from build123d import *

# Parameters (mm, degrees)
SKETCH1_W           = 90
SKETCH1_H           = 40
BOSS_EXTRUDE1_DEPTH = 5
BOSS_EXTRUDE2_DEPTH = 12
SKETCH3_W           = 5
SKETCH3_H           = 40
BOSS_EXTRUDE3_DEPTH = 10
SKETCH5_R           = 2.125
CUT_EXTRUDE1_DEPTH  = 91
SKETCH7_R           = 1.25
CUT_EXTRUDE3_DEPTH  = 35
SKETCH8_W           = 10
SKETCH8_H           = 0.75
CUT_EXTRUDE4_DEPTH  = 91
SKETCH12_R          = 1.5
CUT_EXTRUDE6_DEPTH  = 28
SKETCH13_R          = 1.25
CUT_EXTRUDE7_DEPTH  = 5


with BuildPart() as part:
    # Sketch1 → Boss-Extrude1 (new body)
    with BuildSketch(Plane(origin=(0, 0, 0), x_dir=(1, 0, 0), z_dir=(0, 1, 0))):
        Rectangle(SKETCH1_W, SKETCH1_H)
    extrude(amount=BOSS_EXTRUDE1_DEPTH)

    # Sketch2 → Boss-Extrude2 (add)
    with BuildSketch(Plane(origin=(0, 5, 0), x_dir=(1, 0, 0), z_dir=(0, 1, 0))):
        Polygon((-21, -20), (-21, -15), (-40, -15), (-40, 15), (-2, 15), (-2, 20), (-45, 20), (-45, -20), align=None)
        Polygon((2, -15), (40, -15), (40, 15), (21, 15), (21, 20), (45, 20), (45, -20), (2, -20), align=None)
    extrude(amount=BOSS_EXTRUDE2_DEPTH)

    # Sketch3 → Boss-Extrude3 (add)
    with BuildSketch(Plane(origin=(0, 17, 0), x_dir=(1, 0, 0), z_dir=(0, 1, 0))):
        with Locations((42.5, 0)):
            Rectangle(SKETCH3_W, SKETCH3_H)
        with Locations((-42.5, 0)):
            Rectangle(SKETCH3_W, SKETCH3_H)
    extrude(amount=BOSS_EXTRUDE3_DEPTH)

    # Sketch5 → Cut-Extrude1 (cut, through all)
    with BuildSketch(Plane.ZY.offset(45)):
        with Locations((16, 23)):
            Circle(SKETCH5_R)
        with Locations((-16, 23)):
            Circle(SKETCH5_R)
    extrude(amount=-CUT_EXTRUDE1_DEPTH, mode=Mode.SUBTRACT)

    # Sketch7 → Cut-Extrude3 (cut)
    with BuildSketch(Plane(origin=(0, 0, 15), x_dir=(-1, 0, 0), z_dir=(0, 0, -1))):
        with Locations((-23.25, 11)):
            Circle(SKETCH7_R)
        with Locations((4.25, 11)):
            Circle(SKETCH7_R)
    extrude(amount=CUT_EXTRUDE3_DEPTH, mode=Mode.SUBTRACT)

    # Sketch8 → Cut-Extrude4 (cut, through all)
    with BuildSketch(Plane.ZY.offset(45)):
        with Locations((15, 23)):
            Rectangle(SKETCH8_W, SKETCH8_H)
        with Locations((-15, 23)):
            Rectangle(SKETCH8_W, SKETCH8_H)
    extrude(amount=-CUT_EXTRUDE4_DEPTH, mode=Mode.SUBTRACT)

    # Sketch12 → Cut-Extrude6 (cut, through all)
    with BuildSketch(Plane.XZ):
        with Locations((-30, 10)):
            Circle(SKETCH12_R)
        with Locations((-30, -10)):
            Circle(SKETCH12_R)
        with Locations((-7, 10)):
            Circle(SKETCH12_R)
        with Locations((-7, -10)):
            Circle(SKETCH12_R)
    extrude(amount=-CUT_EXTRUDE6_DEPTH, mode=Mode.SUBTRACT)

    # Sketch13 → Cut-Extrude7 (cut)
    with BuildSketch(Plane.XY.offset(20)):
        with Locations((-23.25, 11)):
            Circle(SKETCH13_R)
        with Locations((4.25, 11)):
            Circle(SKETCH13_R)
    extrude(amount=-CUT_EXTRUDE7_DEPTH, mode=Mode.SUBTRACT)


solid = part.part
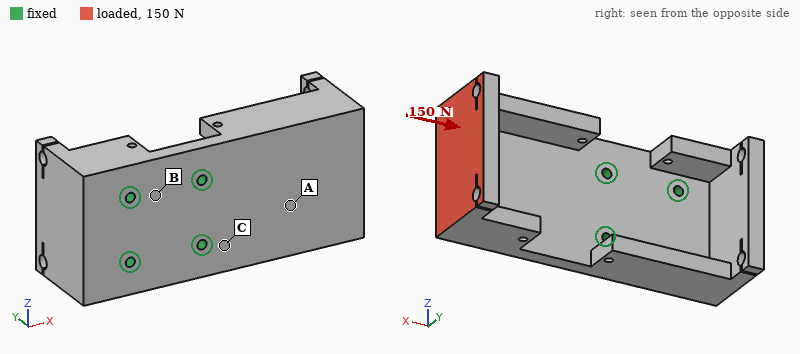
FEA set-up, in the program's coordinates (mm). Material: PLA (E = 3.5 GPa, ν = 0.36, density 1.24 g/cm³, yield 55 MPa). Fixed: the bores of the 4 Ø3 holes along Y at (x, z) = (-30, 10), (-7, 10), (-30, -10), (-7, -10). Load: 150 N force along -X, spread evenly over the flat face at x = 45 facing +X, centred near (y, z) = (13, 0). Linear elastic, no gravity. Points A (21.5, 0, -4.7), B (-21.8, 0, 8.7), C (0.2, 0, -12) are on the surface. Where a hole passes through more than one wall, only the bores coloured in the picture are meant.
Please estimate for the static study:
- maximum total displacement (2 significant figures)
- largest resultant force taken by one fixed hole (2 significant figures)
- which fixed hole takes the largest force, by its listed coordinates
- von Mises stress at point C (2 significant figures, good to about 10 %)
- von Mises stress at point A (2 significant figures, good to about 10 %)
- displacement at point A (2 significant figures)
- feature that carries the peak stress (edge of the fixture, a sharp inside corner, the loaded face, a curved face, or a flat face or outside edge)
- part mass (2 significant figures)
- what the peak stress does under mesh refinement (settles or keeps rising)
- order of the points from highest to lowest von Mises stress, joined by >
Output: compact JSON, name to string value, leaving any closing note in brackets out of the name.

{"maximum total displacement": "1.2 mm", "largest resultant force taken by one fixed hole": "65 N", "which fixed hole takes the largest force, by its listed coordinates": "(-7, 10)", "von Mises stress at point C": "6.8 MPa", "von Mises stress at point A": "3.0 MPa", "displacement at point A": "0.36 mm", "feature that carries the peak stress": "edge of the fixture", "part mass": "41 g", "what the peak stress does under mesh refinement": "keeps rising", "order of the points from highest to lowest von Mises stress, joined by >": "C > A > B"}
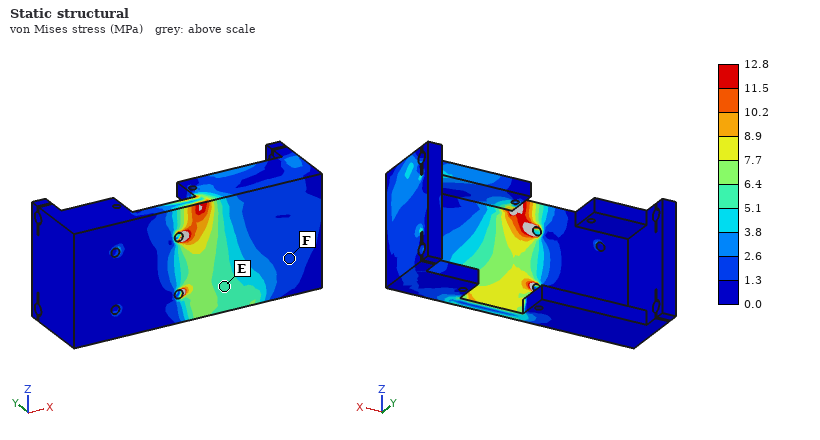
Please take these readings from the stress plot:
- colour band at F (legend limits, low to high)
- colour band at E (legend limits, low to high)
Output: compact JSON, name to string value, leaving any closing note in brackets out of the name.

{"colour band at F": "1.3 to 2.6 MPa", "colour band at E": "5.1 to 6.4 MPa"}
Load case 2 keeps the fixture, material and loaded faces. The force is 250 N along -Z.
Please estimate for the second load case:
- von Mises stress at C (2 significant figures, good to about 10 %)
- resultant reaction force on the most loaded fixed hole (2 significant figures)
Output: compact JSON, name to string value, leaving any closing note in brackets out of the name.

{"von Mises stress at C": "11 MPa", "resultant reaction force on the most loaded fixed hole": "460 N"}
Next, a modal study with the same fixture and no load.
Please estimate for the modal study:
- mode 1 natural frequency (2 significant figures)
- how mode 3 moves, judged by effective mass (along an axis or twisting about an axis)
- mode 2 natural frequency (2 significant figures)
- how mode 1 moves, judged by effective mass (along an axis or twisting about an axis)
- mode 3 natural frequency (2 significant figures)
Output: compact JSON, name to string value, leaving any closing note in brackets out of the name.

{"mode 1 natural frequency": "320 Hz", "how mode 3 moves, judged by effective mass": "along Z", "mode 2 natural frequency": "790 Hz", "how mode 1 moves, judged by effective mass": "along Y", "mode 3 natural frequency": "1800 Hz"}
